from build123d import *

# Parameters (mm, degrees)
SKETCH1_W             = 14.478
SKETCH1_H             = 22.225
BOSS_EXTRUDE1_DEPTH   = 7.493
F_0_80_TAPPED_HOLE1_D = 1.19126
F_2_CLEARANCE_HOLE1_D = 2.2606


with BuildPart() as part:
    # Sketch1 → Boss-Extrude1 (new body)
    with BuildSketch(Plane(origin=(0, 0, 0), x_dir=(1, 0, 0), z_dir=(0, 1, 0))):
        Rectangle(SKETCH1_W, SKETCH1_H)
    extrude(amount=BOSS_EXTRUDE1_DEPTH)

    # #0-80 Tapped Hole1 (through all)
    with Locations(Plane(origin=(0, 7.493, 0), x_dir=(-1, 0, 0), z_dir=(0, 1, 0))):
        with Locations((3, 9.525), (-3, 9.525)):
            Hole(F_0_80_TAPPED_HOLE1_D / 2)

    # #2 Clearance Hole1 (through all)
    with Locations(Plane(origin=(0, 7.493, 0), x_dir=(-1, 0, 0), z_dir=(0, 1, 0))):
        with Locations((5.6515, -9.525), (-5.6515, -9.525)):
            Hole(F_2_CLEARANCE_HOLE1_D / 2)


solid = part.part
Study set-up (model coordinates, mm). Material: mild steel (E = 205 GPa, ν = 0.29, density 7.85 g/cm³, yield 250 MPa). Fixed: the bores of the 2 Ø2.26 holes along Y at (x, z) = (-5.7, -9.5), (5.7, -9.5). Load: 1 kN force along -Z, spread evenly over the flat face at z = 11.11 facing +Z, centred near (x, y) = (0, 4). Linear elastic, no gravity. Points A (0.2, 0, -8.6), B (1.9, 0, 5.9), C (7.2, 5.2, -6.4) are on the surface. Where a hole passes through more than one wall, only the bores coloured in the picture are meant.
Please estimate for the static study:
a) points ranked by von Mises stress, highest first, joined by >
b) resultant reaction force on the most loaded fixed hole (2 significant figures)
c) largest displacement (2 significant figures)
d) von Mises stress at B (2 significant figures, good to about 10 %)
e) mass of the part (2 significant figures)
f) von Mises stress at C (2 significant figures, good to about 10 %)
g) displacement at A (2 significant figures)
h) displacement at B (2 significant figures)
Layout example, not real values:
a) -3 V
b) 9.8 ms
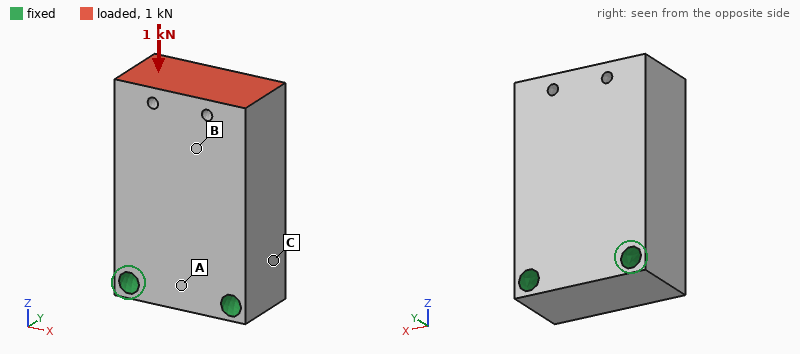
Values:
a) C > B > A
b) 510 N
c) 1.1 µm
d) 9.2 MPa
e) 18 g
f) 12 MPa
g) 0.29 µm
h) 0.76 µm
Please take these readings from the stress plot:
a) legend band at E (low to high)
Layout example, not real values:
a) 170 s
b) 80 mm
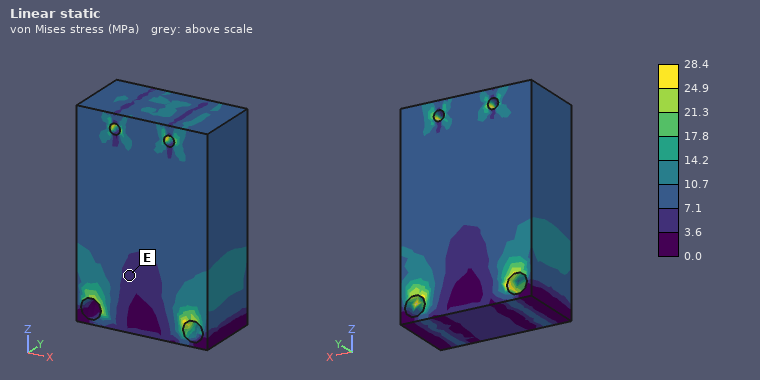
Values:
a) 3.6 to 7.1 MPa
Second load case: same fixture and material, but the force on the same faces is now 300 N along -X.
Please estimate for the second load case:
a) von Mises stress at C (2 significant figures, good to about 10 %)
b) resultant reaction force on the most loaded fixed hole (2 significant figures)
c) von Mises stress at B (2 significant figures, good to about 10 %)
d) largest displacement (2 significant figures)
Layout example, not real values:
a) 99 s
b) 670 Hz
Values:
a) 20 MPa
b) 550 N
c) 7.7 MPa
d) 3.2 µm
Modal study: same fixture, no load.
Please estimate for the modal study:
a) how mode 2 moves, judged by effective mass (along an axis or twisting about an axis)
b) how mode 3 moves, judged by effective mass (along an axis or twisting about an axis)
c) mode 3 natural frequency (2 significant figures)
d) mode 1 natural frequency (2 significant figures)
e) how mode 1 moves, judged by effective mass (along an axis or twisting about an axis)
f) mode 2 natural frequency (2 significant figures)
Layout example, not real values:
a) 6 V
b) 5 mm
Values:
a) along X
b) twisting about Z
c) 32 kHz
d) 12 kHz
e) along Y
f) 23 kHz
